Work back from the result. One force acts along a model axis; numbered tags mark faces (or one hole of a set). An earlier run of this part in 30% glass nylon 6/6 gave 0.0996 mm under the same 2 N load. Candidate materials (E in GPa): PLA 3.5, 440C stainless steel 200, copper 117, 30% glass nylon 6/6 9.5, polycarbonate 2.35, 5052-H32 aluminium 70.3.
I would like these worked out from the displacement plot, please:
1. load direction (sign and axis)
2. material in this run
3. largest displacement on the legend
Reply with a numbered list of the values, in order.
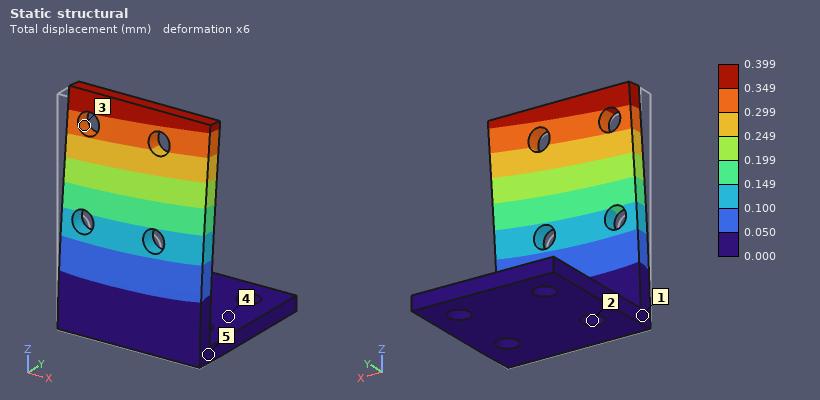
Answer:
1. +Y
2. polycarbonate
3. 0.399 mm
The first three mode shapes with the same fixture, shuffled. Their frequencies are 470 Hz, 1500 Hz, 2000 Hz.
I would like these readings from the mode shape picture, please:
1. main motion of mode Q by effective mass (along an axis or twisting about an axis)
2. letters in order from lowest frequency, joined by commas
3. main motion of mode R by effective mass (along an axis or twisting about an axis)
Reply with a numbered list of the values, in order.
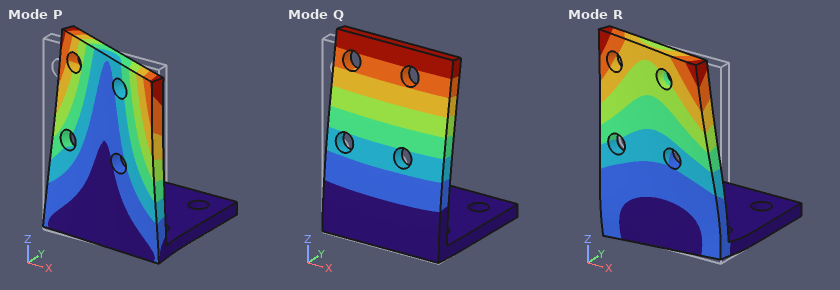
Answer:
1. along Y
2. Q, P, R
3. along X
